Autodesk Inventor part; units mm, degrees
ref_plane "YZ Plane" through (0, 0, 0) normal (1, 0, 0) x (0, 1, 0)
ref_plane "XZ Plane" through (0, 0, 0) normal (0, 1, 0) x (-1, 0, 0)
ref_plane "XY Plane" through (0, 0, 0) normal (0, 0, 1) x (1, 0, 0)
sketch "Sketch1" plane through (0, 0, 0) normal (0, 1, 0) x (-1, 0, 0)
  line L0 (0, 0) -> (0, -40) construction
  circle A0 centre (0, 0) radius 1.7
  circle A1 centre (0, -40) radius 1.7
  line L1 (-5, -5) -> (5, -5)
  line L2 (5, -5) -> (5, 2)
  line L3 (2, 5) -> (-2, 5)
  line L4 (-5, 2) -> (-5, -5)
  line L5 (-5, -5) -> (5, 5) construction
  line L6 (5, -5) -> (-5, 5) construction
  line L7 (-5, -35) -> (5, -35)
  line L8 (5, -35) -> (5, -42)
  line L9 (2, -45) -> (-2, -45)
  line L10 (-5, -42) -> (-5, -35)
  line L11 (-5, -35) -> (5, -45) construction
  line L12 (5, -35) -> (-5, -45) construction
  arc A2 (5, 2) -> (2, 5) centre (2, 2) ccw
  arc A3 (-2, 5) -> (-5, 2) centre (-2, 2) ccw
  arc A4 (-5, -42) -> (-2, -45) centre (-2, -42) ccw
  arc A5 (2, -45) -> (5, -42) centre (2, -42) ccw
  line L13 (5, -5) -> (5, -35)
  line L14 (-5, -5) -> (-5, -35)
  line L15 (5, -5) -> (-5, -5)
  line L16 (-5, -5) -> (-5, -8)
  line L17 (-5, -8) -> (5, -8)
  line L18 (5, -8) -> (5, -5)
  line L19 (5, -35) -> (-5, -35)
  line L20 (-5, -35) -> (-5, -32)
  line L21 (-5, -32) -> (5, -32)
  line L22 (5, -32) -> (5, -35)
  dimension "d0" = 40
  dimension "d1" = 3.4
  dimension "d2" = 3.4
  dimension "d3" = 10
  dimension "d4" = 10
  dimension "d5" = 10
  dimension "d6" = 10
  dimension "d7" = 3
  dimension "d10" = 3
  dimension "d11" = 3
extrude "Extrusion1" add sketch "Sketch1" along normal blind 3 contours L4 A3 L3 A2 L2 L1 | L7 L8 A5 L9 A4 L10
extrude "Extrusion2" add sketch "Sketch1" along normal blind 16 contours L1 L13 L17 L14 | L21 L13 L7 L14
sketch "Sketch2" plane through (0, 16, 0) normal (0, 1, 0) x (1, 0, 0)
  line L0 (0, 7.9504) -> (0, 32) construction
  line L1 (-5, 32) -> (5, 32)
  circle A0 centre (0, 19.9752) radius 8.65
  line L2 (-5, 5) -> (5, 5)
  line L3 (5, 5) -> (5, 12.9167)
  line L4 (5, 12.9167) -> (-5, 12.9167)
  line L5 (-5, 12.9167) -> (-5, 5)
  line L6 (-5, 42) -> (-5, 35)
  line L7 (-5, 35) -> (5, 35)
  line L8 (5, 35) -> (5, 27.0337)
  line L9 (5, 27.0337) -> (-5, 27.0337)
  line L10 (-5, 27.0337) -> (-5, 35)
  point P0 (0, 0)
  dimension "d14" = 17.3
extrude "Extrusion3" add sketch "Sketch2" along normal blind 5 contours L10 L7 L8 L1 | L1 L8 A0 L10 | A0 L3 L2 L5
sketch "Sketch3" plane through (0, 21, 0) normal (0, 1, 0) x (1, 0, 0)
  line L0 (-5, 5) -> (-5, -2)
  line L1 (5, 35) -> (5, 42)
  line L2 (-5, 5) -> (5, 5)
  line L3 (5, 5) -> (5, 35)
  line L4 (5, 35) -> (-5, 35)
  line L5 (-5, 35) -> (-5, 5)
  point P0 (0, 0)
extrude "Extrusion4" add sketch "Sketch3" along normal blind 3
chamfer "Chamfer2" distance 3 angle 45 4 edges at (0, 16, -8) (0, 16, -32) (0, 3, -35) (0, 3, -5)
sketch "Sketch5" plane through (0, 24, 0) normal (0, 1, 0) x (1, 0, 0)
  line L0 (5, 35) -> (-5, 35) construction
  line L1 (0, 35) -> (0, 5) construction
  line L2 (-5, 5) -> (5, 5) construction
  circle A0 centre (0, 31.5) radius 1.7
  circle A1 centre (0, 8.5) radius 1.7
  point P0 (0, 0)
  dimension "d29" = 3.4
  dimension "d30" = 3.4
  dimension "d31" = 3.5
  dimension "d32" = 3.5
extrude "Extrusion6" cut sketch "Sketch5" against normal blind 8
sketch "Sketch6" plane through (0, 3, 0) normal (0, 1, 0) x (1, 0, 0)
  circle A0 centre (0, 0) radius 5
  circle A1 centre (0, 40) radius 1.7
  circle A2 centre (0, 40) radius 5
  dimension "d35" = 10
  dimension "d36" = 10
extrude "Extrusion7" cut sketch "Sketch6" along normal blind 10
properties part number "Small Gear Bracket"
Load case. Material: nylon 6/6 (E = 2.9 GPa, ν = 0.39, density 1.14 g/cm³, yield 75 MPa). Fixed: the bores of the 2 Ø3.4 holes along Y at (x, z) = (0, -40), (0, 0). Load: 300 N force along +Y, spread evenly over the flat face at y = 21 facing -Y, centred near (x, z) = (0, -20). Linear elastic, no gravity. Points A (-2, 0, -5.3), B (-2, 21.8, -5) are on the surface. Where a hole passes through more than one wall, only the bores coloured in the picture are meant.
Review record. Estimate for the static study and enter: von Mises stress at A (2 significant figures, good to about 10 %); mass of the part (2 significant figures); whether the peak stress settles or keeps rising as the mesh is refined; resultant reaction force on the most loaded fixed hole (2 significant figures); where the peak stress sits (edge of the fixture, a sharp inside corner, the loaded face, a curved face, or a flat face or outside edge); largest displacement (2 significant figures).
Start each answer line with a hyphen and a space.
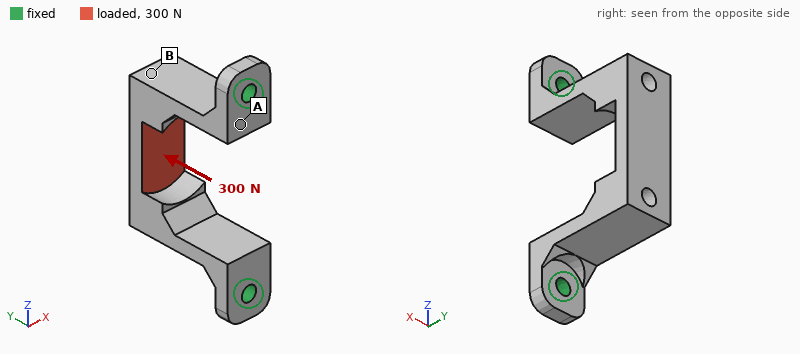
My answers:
- 5.1 MPa
- 3.5 g
- keeps rising
- 170 N
- edge of the fixture
- 0.30 mm
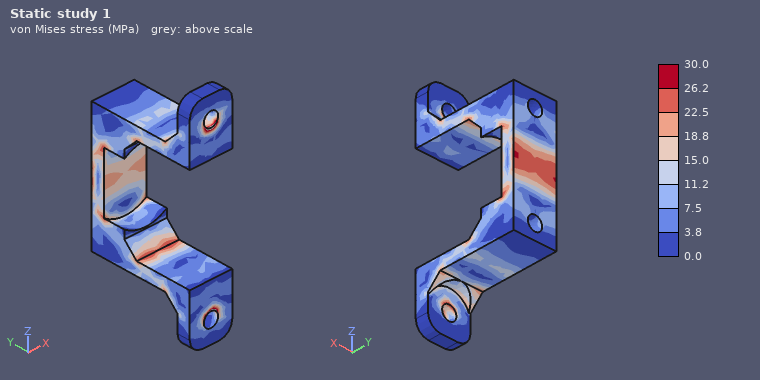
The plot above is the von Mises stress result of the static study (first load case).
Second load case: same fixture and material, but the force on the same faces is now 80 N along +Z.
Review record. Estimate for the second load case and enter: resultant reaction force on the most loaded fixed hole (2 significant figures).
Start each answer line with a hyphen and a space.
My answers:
- 53 N
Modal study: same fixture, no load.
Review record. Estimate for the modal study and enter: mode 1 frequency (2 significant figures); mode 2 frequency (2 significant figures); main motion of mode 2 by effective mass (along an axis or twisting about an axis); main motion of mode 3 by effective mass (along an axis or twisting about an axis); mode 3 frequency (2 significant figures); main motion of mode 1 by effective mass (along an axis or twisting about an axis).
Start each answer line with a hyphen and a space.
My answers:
- 1200 Hz
- 1800 Hz
- along Z
- twisting about Y
- 2300 Hz
- along X
